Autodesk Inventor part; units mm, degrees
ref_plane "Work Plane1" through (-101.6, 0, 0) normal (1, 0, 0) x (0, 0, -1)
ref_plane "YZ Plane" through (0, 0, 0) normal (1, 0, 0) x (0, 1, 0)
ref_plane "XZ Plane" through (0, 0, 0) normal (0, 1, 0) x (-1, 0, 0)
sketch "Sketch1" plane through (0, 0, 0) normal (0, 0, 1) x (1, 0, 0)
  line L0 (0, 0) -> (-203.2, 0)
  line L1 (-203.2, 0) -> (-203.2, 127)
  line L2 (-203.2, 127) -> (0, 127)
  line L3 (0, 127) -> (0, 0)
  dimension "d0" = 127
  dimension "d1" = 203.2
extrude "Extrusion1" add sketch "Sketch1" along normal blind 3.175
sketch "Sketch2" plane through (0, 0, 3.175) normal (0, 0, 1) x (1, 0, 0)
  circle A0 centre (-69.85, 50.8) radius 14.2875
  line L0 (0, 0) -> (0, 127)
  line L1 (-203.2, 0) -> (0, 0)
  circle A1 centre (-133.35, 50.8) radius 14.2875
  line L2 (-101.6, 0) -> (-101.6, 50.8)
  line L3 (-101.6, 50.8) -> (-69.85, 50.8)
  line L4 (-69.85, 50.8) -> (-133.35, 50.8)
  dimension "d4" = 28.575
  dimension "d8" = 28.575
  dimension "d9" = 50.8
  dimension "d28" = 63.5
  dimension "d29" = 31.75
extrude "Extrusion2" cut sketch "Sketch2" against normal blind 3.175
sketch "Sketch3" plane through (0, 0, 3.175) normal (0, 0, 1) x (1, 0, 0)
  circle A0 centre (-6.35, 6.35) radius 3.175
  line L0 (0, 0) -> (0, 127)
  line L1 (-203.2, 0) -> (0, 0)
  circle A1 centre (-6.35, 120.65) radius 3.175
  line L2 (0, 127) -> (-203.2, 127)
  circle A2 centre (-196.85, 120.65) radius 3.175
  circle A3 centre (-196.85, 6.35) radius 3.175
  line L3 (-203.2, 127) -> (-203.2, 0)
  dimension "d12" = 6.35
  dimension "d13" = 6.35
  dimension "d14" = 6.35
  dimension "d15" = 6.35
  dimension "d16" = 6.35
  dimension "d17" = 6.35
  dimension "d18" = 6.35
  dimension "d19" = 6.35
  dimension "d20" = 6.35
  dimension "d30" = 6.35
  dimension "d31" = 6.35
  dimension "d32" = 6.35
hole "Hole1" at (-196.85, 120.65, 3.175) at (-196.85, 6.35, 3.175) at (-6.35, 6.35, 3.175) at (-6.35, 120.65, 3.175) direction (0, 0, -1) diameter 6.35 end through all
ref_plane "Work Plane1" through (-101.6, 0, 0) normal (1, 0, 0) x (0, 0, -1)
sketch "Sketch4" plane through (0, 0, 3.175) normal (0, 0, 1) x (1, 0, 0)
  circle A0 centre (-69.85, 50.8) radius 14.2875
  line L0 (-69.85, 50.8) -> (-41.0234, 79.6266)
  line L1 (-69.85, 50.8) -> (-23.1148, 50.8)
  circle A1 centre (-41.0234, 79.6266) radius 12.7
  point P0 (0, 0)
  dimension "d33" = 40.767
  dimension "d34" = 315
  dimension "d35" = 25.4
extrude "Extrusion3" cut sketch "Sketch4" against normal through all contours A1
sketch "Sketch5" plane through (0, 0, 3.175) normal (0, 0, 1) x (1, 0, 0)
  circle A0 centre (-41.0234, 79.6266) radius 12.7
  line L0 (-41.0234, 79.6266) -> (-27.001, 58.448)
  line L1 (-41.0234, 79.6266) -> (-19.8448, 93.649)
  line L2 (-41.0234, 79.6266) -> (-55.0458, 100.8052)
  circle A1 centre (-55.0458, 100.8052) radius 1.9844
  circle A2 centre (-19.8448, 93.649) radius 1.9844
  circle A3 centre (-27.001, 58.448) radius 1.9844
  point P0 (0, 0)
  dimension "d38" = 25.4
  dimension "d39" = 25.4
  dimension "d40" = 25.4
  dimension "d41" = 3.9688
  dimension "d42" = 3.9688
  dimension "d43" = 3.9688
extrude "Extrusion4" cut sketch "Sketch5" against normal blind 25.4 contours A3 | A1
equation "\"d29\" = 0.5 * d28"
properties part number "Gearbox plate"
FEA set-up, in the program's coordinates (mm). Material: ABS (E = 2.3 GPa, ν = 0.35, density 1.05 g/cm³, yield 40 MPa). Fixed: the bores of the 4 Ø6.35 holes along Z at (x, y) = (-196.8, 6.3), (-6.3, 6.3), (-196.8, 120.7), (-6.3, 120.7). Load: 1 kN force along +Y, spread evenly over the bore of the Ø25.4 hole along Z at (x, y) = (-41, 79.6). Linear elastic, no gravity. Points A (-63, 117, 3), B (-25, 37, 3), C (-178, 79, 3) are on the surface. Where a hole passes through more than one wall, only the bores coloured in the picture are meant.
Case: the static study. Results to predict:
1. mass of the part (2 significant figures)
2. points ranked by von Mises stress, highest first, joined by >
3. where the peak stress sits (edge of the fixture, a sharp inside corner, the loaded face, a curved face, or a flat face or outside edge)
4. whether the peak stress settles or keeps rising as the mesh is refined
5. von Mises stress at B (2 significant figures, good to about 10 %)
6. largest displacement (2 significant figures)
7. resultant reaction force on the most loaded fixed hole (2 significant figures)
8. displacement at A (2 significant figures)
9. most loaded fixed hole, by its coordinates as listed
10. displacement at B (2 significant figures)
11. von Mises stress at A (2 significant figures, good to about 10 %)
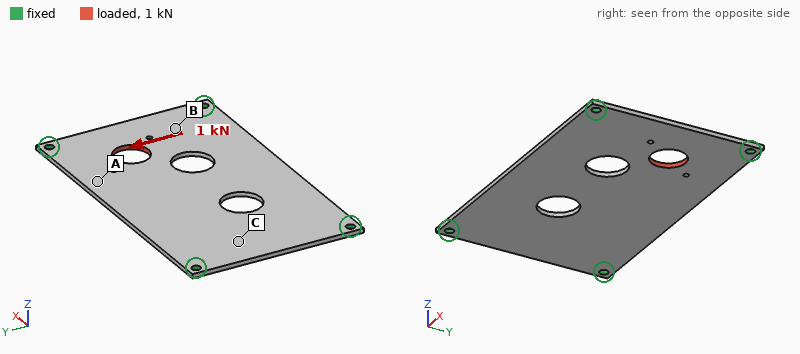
80 g
B > A > C
edge of the fixture
keeps rising
3.7 MPa
0.21 mm
470 N
0.18 mm
(-6.3, 120.7)
0.093 mm
2.0 MPa
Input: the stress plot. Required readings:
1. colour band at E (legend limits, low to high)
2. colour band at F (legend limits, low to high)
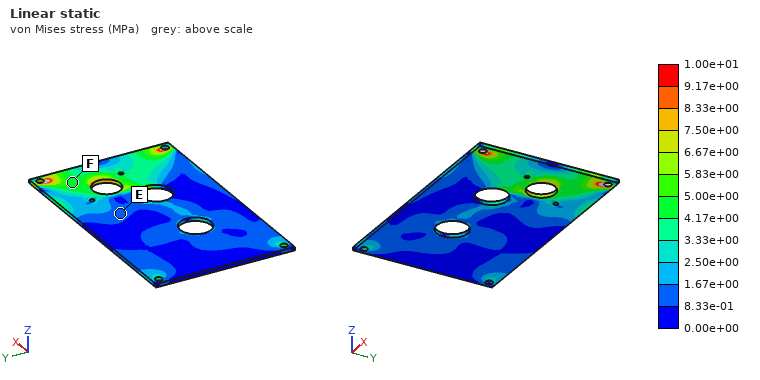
8.33e-01 to 1.67e+00 MPa
4.17e+00 to 5.00e+00 MPa
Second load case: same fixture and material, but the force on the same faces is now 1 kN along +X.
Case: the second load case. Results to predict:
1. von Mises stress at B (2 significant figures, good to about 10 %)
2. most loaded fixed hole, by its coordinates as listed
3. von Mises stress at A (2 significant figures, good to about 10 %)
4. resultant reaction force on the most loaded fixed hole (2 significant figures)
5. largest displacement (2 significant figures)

2.7 MPa
(-6.3, 120.7)
1.4 MPa
440 N
0.21 mm
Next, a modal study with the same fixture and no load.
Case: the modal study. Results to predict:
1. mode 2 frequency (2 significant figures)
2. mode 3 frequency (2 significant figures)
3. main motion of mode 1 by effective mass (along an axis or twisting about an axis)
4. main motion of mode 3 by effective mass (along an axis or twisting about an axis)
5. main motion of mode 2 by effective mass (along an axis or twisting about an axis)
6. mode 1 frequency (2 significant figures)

180 Hz
280 Hz
along Z
twisting about Y
twisting about X
110 Hz
